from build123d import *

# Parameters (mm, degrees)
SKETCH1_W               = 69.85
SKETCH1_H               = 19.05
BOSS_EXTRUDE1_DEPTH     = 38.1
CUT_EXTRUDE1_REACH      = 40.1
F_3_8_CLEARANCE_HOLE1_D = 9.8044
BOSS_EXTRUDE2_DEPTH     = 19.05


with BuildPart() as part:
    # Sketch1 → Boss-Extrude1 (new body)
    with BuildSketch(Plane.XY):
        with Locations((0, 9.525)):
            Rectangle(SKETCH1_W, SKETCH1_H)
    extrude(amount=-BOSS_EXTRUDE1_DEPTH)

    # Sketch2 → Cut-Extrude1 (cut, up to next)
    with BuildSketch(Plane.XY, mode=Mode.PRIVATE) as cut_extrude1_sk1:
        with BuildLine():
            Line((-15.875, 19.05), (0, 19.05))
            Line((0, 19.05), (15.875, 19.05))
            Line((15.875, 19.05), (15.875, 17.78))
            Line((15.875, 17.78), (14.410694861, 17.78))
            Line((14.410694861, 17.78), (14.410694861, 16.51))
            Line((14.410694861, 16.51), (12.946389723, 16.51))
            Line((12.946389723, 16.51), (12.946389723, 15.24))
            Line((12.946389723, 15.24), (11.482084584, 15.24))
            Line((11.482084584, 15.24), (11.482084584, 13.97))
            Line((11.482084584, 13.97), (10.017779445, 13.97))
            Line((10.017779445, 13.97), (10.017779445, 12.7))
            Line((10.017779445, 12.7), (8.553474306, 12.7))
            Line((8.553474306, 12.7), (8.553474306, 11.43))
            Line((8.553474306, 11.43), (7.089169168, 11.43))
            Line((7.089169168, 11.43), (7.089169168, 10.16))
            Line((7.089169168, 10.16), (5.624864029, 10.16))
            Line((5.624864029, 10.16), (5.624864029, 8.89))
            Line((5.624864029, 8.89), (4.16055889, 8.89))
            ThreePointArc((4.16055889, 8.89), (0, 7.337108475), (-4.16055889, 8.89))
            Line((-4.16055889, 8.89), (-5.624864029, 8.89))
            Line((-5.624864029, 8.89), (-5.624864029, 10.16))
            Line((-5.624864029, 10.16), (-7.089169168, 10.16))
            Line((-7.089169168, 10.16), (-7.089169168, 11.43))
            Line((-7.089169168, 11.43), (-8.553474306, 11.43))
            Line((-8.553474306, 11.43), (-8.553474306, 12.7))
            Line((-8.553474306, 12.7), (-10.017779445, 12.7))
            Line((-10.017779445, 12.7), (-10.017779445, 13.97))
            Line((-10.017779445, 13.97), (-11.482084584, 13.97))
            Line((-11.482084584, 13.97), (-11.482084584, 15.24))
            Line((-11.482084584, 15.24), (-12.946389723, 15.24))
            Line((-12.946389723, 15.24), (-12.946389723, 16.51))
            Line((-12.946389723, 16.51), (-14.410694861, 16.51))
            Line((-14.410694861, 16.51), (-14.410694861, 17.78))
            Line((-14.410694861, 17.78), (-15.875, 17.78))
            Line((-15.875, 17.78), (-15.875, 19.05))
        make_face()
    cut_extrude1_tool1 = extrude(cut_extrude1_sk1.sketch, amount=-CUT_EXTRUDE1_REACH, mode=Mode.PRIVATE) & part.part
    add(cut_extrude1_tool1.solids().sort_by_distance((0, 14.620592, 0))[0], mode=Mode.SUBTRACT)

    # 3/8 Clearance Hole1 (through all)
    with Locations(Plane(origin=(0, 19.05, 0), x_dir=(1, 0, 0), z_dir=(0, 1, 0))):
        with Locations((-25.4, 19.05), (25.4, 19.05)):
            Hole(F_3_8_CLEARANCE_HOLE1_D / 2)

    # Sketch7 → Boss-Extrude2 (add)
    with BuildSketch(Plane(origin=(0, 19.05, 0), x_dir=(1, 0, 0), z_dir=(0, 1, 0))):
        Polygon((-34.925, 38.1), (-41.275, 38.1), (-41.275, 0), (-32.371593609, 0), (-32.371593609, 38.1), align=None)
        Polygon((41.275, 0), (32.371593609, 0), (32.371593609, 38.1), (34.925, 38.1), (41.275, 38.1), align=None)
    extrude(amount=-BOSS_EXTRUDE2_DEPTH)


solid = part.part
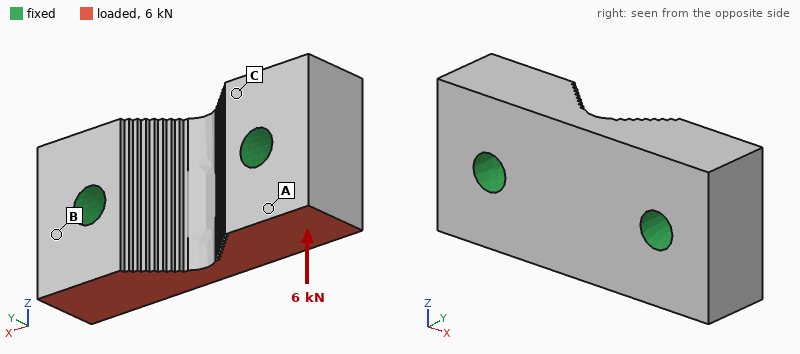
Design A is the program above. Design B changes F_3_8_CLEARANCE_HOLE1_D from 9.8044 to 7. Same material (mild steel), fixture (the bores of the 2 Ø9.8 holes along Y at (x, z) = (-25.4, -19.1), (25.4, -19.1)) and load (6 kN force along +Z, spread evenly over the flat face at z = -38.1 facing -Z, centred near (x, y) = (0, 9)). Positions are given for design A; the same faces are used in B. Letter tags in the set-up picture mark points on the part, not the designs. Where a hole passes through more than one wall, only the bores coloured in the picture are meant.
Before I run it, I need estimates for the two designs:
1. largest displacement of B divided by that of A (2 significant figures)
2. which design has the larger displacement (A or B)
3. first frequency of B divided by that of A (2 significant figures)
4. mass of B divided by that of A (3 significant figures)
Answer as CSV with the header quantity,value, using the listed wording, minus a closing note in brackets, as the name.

quantity,value
largest displacement of B divided by that of A,1.1
which design has the larger displacement,B
first frequency of B divided by that of A,0.84
mass of B divided by that of A,1.03
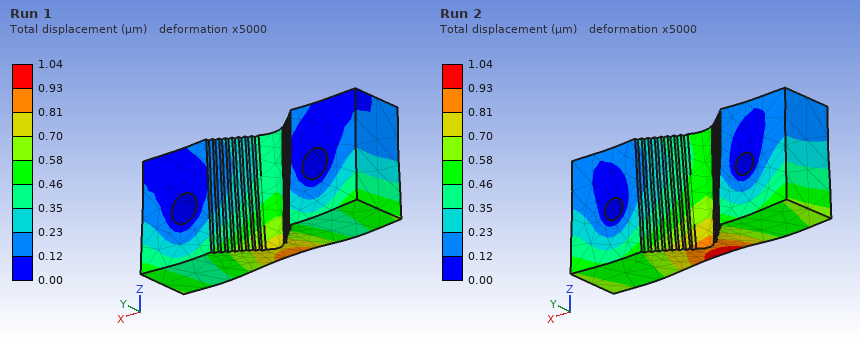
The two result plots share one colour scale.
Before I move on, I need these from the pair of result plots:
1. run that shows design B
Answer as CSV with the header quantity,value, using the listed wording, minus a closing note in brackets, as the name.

quantity,value
run that shows design B,Run 2
